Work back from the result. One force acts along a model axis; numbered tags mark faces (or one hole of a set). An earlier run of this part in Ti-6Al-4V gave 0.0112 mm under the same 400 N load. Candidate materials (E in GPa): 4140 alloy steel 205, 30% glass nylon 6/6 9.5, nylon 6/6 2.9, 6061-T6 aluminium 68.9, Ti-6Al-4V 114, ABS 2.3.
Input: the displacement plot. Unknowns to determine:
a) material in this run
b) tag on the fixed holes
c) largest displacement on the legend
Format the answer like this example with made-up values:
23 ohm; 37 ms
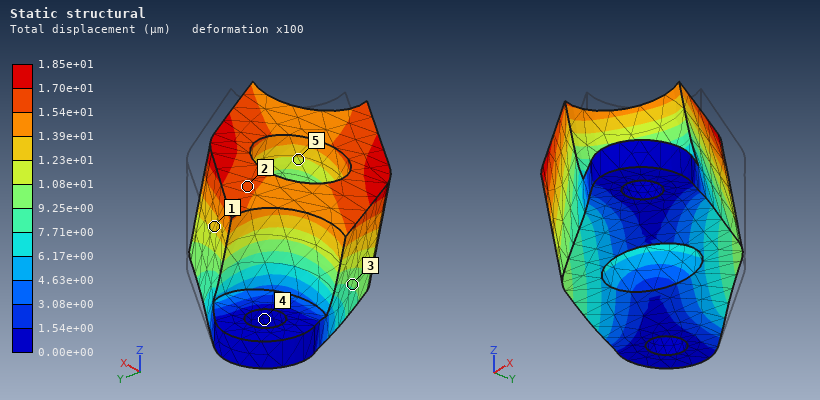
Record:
6061-T6 aluminium; 4; 1.85e+01 µm
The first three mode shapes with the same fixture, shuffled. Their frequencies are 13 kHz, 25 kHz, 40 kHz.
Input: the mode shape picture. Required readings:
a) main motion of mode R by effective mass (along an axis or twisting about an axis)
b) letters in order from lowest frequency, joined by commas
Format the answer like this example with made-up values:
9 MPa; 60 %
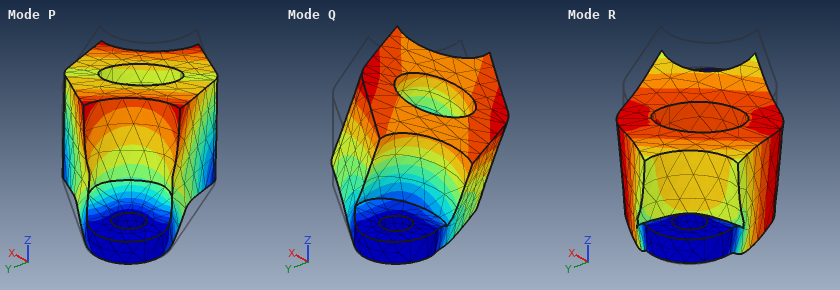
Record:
along Z; Q, R, P
